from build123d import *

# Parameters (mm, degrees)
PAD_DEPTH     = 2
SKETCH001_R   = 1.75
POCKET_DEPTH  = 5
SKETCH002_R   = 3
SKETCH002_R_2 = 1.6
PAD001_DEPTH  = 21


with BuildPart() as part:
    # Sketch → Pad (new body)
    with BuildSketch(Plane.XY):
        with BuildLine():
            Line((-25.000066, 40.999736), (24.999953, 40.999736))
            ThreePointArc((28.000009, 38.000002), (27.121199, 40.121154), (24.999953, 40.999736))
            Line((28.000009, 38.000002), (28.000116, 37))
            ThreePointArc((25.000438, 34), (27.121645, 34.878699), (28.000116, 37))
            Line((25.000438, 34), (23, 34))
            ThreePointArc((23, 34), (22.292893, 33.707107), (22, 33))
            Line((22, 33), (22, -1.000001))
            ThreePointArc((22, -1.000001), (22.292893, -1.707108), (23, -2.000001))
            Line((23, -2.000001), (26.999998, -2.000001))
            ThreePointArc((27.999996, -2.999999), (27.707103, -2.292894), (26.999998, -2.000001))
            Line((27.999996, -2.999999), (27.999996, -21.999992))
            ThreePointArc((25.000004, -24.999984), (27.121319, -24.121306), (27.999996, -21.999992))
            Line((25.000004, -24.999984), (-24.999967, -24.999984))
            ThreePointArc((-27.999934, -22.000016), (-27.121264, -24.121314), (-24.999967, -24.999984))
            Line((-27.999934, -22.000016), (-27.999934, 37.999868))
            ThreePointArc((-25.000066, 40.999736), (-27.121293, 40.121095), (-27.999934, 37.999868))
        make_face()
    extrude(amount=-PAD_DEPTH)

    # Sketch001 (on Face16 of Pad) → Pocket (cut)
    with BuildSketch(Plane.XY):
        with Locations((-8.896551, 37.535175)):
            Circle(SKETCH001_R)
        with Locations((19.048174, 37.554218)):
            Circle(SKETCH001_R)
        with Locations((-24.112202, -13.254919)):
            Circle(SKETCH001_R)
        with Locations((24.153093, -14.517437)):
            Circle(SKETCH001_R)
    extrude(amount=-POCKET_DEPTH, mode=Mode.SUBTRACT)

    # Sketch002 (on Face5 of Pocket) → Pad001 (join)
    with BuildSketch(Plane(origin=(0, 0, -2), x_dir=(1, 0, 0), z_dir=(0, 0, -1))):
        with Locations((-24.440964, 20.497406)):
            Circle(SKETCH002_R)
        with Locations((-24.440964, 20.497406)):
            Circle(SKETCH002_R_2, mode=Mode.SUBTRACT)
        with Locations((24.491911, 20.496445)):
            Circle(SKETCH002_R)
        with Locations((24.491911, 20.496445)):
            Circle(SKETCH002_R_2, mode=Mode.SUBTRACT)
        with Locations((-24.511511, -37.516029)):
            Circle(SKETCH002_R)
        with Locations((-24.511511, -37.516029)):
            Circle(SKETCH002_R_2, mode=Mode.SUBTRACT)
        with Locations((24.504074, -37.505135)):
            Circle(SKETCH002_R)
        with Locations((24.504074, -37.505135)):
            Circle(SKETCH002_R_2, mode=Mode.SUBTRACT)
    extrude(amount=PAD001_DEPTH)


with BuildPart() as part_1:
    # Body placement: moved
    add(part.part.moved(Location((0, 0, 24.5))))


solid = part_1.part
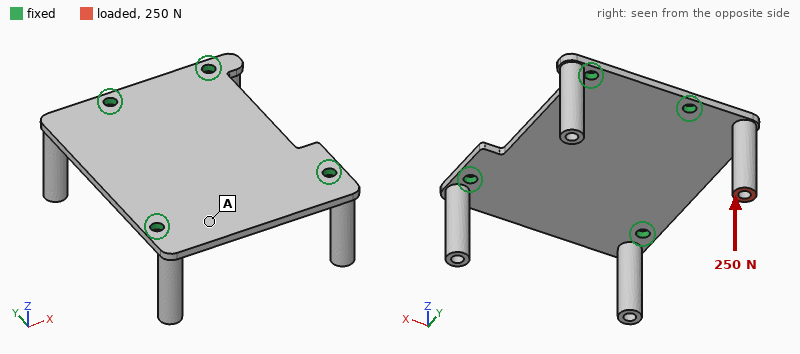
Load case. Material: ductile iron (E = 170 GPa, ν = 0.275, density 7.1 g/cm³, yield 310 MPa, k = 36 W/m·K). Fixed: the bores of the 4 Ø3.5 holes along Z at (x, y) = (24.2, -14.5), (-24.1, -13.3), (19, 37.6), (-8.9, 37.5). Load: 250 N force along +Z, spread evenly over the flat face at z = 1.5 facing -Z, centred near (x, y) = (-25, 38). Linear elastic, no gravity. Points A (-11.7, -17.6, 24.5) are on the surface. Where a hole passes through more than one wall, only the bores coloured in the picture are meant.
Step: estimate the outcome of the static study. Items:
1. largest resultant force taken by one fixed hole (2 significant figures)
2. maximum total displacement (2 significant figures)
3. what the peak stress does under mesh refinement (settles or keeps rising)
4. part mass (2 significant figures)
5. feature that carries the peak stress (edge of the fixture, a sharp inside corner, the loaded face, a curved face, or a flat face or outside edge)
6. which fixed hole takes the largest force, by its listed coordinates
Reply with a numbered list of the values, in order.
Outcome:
1. 270 N
2. 0.32 mm
3. keeps rising
4. 61 g
5. edge of the fixture
6. (-8.9, 37.5)
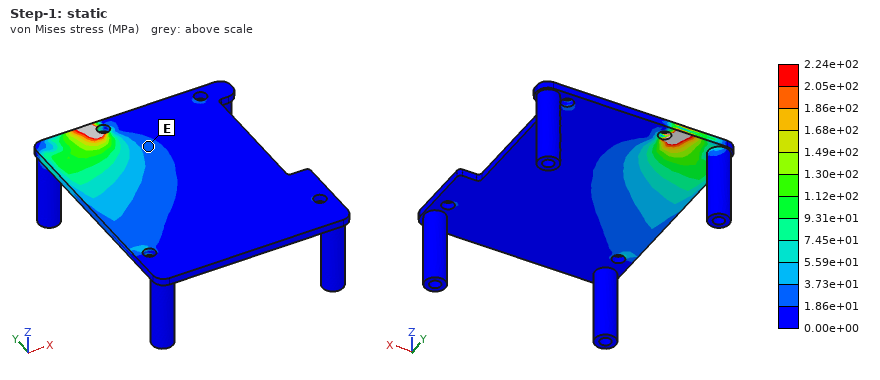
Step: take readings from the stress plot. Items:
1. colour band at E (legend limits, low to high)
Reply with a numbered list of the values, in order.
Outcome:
1. 1.86e+01 to 3.73e+01 MPa
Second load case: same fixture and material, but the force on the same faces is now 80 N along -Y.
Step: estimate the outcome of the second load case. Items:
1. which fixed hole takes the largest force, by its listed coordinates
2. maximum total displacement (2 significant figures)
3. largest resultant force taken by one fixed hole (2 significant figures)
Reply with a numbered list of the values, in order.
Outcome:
1. (-8.9, 37.5)
2. 0.21 mm
3. 53 N
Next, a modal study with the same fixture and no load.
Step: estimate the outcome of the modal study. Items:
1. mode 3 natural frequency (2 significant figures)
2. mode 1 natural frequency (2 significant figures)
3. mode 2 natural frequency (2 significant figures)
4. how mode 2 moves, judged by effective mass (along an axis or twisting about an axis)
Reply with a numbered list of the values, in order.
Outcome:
1. 3300 Hz
2. 2100 Hz
3. 2700 Hz
4. along Z
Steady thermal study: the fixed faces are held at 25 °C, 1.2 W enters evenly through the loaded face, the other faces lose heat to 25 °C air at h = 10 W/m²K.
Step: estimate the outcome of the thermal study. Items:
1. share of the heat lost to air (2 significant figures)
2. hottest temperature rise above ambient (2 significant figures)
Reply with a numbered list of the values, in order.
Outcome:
1. 24 %
2. 45 K
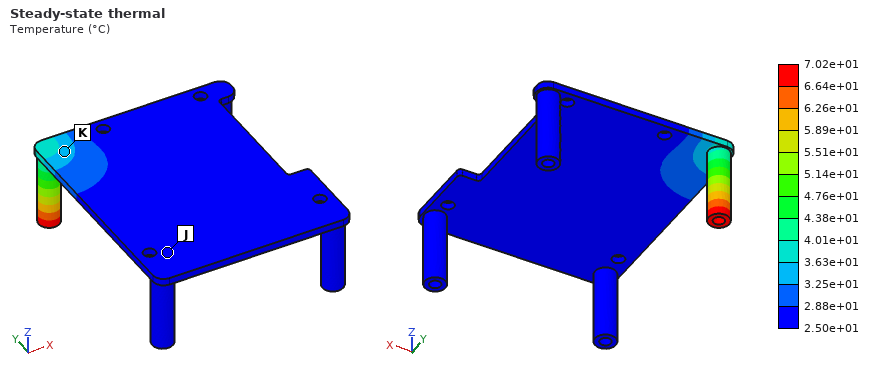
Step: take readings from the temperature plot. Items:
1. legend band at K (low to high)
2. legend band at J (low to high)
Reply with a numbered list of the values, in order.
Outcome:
1. 3.25e+01 to 3.63e+01 °C
2. 2.50e+01 to 2.88e+01 °C
